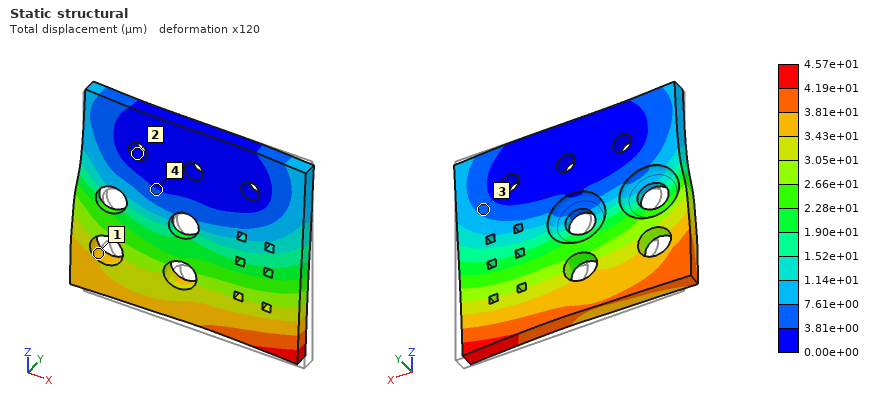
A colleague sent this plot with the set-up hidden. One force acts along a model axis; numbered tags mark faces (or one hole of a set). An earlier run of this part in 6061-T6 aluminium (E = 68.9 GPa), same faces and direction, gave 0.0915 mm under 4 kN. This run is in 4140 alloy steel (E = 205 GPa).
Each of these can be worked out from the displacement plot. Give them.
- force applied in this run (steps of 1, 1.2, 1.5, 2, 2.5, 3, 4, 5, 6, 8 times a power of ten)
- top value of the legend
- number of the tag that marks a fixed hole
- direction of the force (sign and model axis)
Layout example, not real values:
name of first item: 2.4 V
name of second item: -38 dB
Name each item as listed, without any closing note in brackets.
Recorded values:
force applied in this run: 6 kN
top value of the legend: 4.57e+01 µm
number of the tag that marks a fixed hole: 2
direction of the force: -X
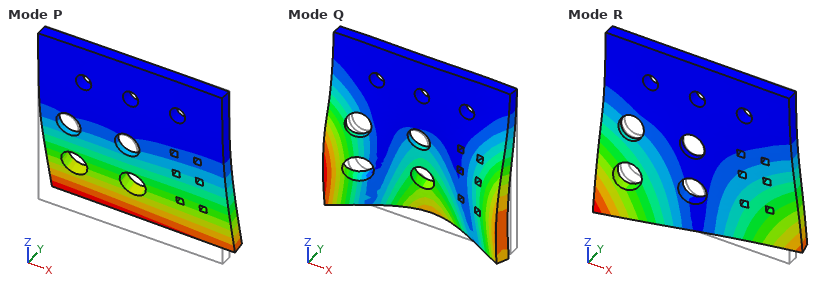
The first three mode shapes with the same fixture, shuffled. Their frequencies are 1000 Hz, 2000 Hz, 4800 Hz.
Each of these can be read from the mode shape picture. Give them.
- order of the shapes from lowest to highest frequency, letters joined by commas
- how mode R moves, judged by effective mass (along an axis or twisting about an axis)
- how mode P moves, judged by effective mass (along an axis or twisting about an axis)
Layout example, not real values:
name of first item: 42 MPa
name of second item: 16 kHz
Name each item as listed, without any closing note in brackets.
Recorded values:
order of the shapes from lowest to highest frequency, letters joined by commas: P, R, Q
how mode R moves, judged by effective mass: twisting about Z
how mode P moves, judged by effective mass: along Y
